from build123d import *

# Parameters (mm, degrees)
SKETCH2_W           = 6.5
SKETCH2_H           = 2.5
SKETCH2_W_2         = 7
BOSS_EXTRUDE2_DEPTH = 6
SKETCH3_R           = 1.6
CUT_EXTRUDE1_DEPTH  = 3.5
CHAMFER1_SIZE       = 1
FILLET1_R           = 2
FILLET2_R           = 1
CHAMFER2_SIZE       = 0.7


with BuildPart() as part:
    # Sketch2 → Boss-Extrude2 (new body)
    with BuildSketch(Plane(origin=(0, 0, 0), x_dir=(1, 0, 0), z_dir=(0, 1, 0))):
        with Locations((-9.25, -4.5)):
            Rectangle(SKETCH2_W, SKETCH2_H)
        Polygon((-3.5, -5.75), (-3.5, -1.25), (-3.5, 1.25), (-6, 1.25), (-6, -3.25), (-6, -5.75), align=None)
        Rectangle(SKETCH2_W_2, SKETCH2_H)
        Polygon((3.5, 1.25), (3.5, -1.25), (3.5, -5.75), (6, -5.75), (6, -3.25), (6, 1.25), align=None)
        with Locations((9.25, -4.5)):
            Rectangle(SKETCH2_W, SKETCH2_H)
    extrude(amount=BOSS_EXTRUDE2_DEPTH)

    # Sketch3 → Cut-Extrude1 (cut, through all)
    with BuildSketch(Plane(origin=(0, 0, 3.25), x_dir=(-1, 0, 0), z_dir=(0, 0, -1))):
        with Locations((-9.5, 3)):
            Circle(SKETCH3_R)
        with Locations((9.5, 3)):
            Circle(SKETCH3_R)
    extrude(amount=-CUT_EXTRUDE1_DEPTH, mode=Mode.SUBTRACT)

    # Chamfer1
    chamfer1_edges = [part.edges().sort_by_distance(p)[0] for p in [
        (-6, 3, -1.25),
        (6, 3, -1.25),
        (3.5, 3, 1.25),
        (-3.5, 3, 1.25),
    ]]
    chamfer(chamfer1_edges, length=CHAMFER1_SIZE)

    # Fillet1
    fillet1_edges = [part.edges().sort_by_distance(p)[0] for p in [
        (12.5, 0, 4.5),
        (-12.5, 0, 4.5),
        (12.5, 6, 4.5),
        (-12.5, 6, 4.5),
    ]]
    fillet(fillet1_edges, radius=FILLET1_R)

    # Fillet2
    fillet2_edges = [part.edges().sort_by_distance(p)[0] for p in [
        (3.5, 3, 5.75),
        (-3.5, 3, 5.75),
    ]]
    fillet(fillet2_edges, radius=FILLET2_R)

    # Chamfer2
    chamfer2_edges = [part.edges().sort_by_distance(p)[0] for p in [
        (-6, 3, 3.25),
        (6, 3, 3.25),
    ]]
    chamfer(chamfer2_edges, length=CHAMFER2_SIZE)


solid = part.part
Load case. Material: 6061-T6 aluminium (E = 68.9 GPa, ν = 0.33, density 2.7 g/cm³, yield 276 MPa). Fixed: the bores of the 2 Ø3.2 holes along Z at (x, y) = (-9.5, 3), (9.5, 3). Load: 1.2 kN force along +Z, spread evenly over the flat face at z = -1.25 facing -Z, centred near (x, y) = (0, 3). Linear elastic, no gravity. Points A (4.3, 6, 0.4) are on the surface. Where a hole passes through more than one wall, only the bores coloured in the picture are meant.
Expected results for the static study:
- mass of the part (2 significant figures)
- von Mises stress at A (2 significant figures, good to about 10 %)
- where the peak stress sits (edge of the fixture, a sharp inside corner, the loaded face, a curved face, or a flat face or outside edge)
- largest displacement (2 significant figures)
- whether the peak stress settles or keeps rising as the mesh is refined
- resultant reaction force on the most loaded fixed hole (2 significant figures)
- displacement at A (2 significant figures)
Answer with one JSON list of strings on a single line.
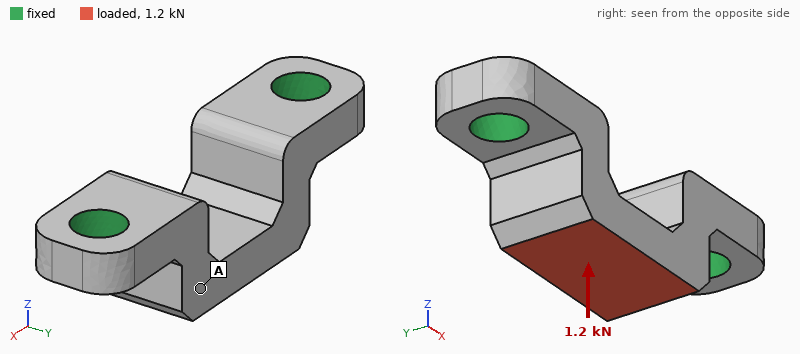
["1.2 g", "38 MPa", "edge of the fixture", "16 µm", "keeps rising", "770 N", "11 µm"]
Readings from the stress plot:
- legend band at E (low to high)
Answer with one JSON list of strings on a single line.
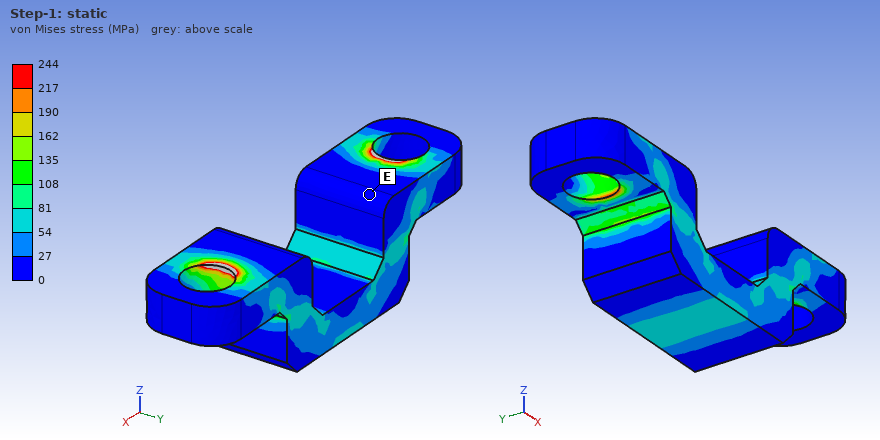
["0 to 27 MPa"]
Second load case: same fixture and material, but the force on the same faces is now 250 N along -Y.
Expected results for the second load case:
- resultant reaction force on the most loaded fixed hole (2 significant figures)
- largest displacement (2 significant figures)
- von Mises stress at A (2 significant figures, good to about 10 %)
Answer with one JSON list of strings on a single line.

["130 N", "23 µm", "15 MPa"]
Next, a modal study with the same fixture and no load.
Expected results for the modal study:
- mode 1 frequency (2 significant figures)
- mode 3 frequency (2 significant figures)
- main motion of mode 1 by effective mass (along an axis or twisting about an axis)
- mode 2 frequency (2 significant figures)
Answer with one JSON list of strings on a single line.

["28 kHz", "57 kHz", "along Y", "56 kHz"]
